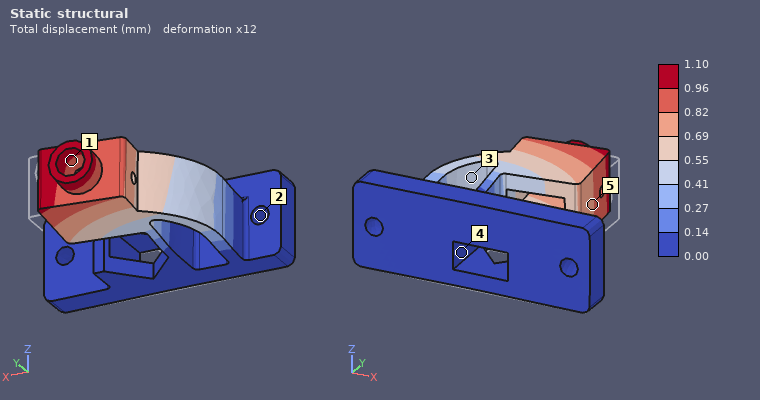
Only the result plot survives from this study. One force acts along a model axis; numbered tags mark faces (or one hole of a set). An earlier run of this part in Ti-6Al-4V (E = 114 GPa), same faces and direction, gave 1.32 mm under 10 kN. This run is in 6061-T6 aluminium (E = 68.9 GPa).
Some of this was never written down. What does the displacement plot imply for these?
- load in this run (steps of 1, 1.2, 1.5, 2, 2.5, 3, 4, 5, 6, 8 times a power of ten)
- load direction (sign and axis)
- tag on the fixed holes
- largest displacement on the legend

5 kN
-X
2
1.10 mm
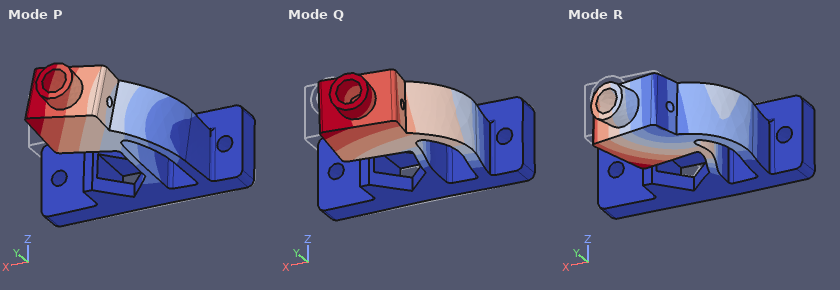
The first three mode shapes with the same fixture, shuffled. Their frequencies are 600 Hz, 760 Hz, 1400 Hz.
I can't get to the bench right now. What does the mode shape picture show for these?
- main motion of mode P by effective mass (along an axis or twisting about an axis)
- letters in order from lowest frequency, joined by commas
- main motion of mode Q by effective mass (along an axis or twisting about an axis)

along Z
P, Q, R
along X
